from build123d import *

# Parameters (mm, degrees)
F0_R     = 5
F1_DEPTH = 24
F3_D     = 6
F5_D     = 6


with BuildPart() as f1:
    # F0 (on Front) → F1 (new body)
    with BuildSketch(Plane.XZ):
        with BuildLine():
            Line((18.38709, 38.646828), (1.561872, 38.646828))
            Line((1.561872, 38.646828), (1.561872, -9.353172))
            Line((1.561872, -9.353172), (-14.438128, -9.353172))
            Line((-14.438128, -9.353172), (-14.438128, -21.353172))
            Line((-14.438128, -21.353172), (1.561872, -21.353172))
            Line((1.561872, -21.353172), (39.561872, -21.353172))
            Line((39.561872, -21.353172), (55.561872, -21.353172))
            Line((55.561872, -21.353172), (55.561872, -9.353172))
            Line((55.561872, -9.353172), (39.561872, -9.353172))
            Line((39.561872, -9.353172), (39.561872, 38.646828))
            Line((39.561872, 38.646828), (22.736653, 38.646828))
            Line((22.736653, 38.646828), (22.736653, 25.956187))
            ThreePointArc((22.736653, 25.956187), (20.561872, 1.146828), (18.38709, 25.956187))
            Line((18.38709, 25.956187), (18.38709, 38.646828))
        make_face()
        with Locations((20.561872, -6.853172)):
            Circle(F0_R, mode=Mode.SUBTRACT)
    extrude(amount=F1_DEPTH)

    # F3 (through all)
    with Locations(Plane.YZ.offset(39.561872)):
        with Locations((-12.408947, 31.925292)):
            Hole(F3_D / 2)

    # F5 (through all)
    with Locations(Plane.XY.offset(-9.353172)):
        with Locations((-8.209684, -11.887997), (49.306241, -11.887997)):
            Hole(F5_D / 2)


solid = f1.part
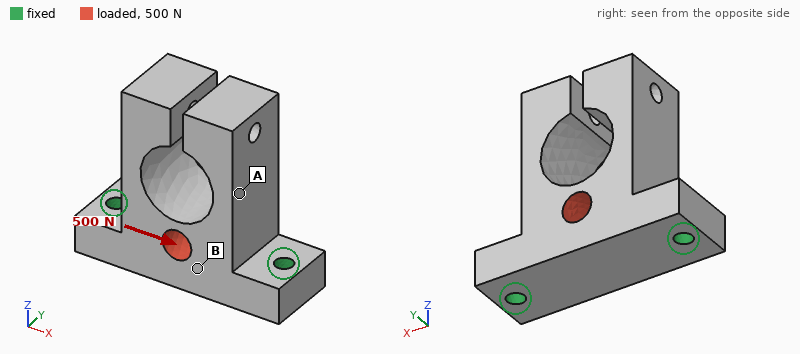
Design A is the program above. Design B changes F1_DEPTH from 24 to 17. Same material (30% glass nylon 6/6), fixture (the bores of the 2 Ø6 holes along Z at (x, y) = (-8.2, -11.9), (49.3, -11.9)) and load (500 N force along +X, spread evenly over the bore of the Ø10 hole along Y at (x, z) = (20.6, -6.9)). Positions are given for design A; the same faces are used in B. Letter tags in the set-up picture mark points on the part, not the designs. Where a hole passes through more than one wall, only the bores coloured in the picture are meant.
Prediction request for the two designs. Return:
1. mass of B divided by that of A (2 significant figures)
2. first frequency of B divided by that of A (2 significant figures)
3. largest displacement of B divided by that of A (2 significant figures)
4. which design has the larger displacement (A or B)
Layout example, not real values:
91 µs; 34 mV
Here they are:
0.70; 0.88; 1.4; B
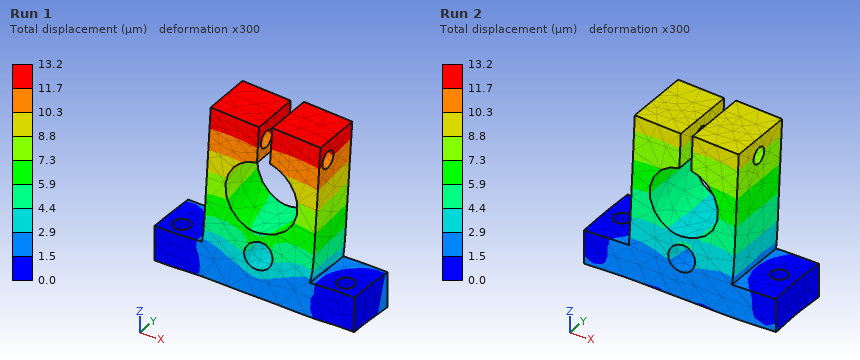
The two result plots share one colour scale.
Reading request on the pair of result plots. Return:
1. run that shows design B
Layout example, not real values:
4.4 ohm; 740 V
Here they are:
Run 1
